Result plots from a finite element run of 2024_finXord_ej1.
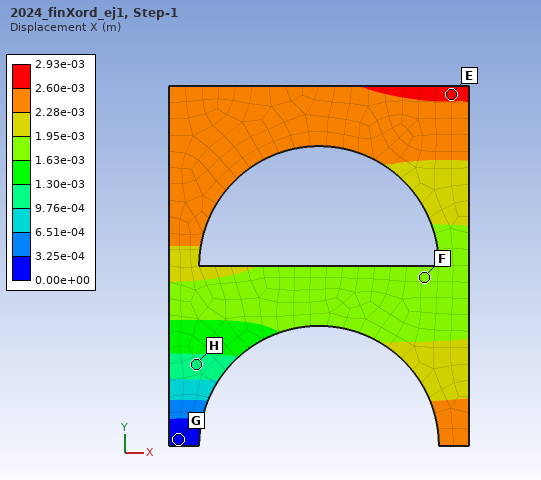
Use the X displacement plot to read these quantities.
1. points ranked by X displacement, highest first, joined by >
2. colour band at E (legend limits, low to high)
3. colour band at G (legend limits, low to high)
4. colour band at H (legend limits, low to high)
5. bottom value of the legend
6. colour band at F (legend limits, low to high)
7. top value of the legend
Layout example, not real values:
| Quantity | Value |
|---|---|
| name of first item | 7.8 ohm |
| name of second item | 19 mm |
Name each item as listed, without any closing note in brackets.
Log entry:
| Quantity | Value |
|---|---|
| points ranked by X displacement, highest first, joined by > | E > F > H > G |
| colour band at E | 2.60e-03 to 2.93e-03 m |
| colour band at G | 0.00e+00 to 3.25e-04 m |
| colour band at H | 9.76e-04 to 1.30e-03 m |
| bottom value of the legend | 0.00e+00 m |
| colour band at F | 1.63e-03 to 1.95e-03 m |
| top value of the legend | 2.93e-03 m |
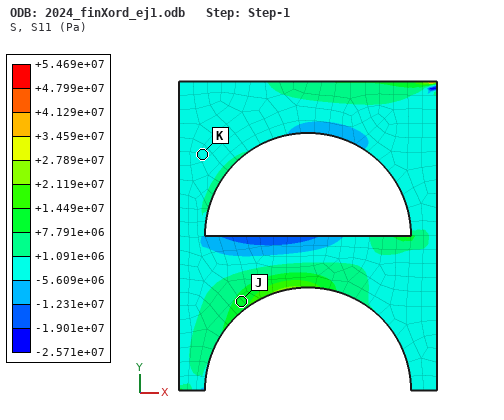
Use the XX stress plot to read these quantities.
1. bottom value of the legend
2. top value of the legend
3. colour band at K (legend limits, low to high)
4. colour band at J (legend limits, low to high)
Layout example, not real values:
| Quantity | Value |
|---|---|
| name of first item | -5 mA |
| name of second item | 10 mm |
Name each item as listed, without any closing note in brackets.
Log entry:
| Quantity | Value |
|---|---|
| bottom value of the legend | -2.571e+07 Pa |
| top value of the legend | +5.469e+07 Pa |
| colour band at K | -5.609e+06 to +1.091e+06 Pa |
| colour band at J | +7.791e+06 to +1.449e+07 Pa |
